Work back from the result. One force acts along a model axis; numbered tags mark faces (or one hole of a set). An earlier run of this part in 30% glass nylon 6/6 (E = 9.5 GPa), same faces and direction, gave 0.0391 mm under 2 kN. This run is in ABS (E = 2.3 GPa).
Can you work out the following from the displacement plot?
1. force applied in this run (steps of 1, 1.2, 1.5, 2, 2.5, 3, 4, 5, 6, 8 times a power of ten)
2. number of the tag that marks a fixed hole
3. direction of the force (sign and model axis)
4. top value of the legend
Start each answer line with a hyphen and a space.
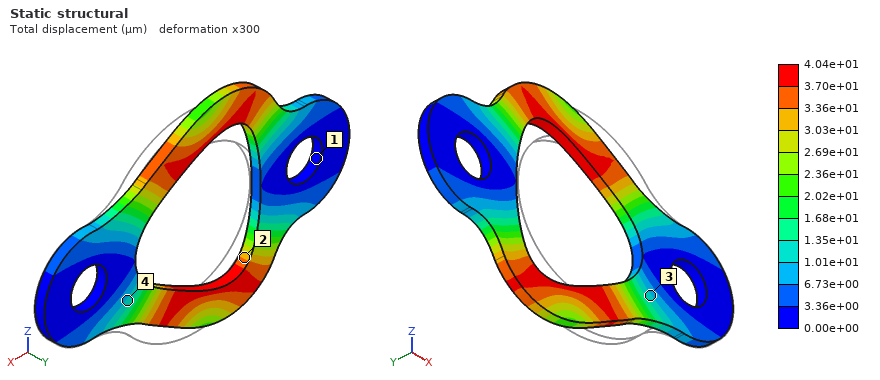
- 500 N
- 1
- -X
- 4.04e+01 µm
